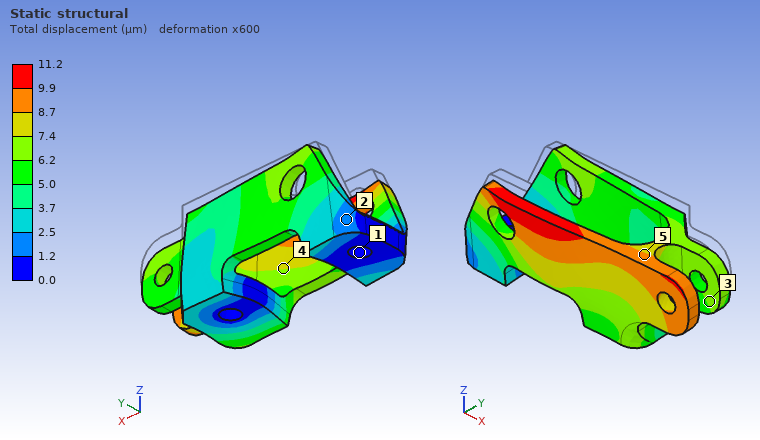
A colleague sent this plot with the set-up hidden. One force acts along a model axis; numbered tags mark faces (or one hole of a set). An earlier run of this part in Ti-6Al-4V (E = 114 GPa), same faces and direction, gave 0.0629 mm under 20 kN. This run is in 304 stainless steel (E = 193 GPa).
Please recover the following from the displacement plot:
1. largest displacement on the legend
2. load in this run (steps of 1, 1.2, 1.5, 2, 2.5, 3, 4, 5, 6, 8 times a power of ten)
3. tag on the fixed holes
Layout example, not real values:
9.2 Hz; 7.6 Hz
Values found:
11.2 µm; 6 kN; 1
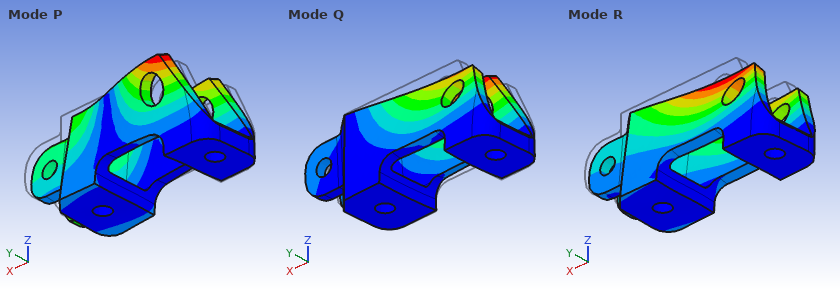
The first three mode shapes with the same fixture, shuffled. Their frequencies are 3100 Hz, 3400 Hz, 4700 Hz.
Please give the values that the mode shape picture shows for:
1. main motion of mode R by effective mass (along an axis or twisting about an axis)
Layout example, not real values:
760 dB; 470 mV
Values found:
along Y
